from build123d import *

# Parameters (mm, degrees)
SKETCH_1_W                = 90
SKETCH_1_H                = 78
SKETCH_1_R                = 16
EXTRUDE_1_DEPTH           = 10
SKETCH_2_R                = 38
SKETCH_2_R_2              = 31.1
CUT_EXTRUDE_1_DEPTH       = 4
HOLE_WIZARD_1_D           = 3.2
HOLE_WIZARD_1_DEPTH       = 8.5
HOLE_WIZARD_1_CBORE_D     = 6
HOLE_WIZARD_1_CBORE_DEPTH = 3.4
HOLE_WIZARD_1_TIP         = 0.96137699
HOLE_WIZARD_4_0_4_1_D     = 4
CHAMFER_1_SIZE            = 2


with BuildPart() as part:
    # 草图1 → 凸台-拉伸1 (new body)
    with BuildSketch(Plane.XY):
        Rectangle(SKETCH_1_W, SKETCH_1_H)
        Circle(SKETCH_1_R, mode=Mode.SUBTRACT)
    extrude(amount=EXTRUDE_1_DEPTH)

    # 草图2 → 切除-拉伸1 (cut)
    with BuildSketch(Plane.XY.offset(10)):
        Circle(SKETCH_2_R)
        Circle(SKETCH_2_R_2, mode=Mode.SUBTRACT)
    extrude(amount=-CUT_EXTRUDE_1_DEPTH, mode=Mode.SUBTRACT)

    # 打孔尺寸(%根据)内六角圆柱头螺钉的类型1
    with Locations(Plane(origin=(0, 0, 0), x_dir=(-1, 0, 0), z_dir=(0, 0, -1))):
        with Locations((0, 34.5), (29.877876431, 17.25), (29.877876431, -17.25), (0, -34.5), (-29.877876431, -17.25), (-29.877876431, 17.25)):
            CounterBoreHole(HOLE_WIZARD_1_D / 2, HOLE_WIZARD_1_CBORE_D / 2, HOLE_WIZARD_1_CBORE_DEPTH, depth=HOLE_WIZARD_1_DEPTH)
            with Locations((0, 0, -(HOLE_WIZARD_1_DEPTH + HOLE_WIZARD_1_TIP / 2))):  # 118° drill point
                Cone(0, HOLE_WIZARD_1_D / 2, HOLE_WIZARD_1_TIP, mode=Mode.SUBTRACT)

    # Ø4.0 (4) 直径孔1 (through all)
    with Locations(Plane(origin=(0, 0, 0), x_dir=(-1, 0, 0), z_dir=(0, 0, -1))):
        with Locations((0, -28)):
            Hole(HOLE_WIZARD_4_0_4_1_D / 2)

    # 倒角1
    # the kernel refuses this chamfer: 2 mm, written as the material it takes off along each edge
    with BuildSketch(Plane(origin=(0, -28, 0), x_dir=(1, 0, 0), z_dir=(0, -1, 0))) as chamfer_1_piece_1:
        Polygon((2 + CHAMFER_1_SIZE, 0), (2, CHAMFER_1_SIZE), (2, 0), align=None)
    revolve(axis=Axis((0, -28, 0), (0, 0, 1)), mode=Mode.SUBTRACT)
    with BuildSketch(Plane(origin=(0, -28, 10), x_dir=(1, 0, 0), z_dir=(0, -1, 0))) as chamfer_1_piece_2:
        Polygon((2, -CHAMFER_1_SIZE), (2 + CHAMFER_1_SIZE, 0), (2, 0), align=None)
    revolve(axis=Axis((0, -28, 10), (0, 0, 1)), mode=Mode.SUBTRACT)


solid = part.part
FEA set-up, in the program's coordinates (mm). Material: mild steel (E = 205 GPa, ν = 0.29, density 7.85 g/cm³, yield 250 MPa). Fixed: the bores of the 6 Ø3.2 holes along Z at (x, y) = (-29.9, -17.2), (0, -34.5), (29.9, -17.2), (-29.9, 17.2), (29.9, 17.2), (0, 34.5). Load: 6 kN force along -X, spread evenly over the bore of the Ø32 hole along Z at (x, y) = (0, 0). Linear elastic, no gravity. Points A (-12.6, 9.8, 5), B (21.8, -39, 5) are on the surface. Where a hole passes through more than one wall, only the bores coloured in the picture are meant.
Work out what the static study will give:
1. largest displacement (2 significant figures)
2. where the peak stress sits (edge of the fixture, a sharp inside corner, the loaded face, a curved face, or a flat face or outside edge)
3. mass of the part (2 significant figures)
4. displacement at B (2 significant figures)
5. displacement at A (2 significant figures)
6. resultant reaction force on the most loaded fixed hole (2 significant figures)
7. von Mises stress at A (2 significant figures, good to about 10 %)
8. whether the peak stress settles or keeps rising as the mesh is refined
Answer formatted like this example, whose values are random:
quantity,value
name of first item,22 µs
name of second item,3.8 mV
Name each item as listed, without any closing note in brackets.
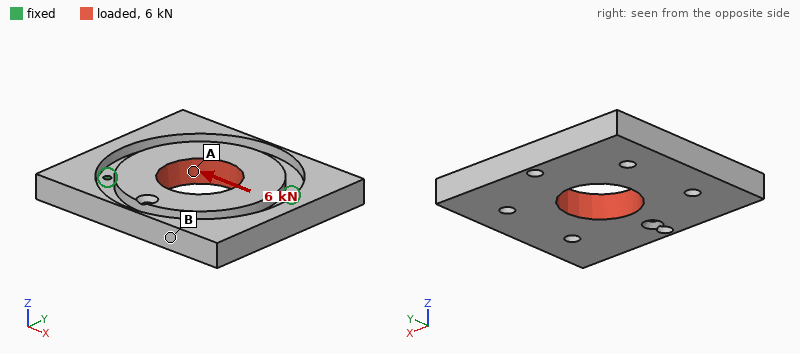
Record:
quantity,value
largest displacement,1.5 µm
where the peak stress sits,edge of the fixture
mass of the part,430 g
displacement at B,0.61 µm
displacement at A,1.4 µm
resultant reaction force on the most loaded fixed hole,1.2 kN
von Mises stress at A,8.2 MPa
whether the peak stress settles or keeps rising as the mesh is refined,keeps rising
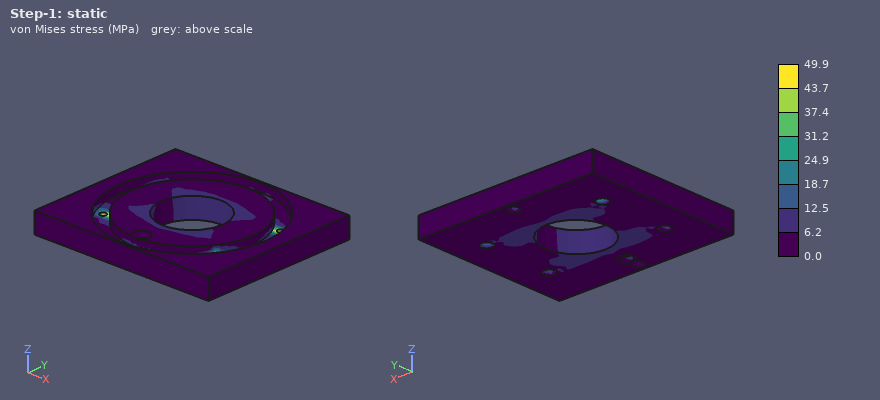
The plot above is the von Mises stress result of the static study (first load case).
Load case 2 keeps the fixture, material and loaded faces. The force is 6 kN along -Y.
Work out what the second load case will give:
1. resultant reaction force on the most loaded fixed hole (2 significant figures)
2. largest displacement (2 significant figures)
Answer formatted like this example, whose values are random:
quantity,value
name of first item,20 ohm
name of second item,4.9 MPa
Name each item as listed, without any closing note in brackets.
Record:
quantity,value
resultant reaction force on the most loaded fixed hole,1.2 kN
largest displacement,1.8 µm
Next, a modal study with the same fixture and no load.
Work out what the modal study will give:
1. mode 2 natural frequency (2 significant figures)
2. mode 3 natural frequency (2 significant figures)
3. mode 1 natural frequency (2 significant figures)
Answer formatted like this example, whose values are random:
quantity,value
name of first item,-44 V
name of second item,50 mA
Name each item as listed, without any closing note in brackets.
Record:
quantity,value
mode 2 natural frequency,7500 Hz
mode 3 natural frequency,7600 Hz
mode 1 natural frequency,7000 Hz
